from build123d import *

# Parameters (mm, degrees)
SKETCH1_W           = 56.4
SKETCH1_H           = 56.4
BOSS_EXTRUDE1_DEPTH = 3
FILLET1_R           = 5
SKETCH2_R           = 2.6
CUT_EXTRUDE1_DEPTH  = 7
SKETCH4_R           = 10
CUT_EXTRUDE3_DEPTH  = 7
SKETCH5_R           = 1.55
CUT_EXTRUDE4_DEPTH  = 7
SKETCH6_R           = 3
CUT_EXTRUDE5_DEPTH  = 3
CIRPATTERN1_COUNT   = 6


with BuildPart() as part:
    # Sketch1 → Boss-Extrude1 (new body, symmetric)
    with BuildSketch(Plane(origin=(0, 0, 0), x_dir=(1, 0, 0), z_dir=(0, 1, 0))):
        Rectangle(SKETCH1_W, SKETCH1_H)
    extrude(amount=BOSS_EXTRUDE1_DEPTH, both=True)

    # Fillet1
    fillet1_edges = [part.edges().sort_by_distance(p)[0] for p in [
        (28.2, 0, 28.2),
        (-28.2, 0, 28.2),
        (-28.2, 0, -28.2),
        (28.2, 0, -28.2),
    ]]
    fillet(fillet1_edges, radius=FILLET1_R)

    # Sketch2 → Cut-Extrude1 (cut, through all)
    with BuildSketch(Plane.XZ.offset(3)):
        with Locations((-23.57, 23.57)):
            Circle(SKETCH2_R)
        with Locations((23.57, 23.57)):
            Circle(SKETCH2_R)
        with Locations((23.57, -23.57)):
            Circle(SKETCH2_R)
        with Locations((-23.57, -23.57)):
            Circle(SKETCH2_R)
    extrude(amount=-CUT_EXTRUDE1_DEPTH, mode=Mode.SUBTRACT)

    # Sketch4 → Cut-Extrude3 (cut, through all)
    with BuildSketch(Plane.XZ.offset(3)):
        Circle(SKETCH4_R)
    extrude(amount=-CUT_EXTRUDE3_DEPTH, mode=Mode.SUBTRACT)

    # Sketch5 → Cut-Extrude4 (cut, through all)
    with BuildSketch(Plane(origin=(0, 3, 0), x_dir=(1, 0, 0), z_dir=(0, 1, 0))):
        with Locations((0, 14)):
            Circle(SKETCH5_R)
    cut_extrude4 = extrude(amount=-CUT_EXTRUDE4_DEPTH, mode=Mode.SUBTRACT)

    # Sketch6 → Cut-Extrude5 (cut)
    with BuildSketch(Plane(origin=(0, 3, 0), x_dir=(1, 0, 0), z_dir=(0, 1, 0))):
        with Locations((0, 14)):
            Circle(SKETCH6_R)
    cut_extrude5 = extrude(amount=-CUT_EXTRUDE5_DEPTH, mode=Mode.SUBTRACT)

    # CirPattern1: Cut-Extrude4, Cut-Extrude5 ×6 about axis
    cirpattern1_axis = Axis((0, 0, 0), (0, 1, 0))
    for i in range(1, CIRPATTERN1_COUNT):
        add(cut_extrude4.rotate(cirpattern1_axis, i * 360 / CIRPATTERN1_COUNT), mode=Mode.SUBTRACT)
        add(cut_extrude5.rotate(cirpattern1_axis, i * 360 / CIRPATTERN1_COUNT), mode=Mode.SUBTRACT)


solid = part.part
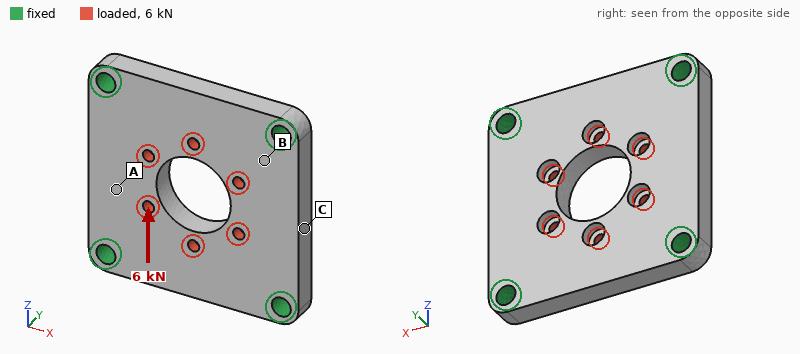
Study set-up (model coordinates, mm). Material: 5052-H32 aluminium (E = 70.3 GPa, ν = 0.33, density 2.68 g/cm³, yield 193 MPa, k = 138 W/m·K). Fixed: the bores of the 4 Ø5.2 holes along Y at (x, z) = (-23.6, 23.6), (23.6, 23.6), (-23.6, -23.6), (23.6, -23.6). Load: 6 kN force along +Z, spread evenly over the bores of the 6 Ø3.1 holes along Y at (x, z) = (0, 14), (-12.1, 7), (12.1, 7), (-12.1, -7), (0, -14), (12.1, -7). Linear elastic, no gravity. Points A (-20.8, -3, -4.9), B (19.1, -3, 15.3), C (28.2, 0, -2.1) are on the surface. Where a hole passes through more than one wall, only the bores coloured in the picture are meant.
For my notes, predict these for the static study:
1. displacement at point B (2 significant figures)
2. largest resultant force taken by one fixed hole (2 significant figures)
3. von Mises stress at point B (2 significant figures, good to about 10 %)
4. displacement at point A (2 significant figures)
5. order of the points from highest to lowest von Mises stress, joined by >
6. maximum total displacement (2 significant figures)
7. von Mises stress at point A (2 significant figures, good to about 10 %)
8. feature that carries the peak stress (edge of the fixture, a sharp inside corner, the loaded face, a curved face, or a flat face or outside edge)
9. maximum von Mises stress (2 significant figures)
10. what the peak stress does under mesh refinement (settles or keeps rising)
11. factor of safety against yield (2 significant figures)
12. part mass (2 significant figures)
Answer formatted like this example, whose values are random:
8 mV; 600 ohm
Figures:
2.9 µm; 1.6 kN; 22 MPa; 3.6 µm; B > A > C; 12 µm; 13 MPa; the loaded face; 70 MPa; settles; 2.8; 43 g
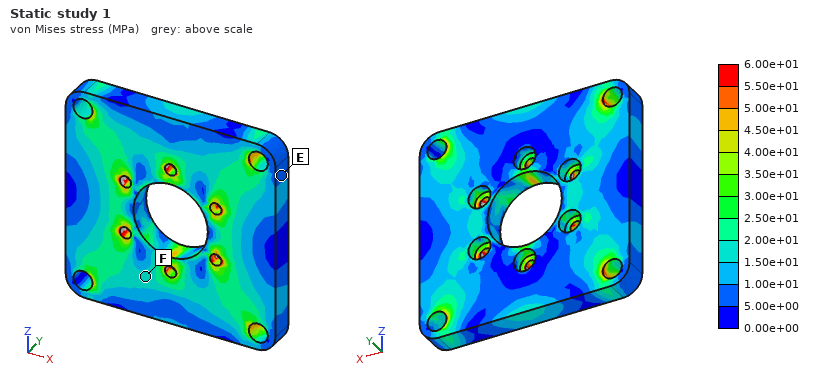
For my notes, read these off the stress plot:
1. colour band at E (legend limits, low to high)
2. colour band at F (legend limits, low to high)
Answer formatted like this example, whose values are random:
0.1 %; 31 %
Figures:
5.00e+00 to 1.00e+01 MPa; 1.50e+01 to 2.00e+01 MPa
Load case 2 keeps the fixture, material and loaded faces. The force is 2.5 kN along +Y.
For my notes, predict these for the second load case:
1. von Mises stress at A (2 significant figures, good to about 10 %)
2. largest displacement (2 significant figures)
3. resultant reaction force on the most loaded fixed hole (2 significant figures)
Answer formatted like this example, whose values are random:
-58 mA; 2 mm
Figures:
28 MPa; 56 µm; 640 N
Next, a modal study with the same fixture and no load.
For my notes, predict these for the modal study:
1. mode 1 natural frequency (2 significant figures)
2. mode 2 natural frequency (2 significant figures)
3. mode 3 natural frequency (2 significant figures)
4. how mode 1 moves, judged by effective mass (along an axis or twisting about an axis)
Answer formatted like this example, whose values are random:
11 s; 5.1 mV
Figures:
10000 Hz; 14 kHz; 15 kHz; along Y
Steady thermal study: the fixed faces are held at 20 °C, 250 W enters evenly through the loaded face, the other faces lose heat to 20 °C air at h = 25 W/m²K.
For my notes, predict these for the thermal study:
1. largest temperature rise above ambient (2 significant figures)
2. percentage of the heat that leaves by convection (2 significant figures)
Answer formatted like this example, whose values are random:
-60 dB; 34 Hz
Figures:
87 K; 3.1 %
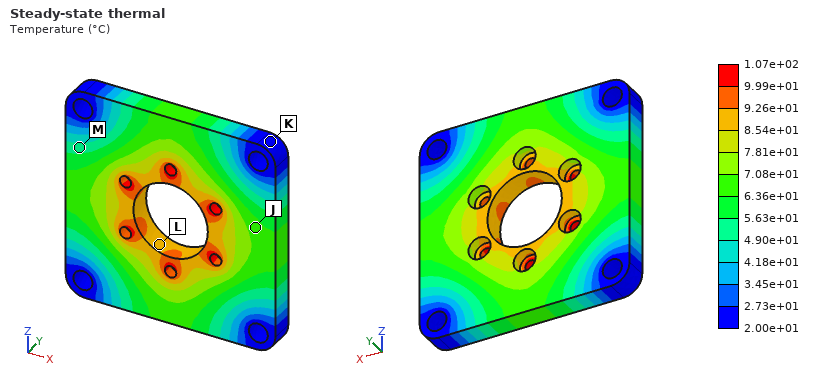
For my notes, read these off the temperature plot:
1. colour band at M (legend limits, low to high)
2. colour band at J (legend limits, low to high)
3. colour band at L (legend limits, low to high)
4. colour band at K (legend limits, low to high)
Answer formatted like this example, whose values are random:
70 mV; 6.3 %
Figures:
4.90e+01 to 5.63e+01 °C; 6.36e+01 to 7.08e+01 °C; 8.54e+01 to 9.26e+01 °C; 2.00e+01 to 2.73e+01 °C
